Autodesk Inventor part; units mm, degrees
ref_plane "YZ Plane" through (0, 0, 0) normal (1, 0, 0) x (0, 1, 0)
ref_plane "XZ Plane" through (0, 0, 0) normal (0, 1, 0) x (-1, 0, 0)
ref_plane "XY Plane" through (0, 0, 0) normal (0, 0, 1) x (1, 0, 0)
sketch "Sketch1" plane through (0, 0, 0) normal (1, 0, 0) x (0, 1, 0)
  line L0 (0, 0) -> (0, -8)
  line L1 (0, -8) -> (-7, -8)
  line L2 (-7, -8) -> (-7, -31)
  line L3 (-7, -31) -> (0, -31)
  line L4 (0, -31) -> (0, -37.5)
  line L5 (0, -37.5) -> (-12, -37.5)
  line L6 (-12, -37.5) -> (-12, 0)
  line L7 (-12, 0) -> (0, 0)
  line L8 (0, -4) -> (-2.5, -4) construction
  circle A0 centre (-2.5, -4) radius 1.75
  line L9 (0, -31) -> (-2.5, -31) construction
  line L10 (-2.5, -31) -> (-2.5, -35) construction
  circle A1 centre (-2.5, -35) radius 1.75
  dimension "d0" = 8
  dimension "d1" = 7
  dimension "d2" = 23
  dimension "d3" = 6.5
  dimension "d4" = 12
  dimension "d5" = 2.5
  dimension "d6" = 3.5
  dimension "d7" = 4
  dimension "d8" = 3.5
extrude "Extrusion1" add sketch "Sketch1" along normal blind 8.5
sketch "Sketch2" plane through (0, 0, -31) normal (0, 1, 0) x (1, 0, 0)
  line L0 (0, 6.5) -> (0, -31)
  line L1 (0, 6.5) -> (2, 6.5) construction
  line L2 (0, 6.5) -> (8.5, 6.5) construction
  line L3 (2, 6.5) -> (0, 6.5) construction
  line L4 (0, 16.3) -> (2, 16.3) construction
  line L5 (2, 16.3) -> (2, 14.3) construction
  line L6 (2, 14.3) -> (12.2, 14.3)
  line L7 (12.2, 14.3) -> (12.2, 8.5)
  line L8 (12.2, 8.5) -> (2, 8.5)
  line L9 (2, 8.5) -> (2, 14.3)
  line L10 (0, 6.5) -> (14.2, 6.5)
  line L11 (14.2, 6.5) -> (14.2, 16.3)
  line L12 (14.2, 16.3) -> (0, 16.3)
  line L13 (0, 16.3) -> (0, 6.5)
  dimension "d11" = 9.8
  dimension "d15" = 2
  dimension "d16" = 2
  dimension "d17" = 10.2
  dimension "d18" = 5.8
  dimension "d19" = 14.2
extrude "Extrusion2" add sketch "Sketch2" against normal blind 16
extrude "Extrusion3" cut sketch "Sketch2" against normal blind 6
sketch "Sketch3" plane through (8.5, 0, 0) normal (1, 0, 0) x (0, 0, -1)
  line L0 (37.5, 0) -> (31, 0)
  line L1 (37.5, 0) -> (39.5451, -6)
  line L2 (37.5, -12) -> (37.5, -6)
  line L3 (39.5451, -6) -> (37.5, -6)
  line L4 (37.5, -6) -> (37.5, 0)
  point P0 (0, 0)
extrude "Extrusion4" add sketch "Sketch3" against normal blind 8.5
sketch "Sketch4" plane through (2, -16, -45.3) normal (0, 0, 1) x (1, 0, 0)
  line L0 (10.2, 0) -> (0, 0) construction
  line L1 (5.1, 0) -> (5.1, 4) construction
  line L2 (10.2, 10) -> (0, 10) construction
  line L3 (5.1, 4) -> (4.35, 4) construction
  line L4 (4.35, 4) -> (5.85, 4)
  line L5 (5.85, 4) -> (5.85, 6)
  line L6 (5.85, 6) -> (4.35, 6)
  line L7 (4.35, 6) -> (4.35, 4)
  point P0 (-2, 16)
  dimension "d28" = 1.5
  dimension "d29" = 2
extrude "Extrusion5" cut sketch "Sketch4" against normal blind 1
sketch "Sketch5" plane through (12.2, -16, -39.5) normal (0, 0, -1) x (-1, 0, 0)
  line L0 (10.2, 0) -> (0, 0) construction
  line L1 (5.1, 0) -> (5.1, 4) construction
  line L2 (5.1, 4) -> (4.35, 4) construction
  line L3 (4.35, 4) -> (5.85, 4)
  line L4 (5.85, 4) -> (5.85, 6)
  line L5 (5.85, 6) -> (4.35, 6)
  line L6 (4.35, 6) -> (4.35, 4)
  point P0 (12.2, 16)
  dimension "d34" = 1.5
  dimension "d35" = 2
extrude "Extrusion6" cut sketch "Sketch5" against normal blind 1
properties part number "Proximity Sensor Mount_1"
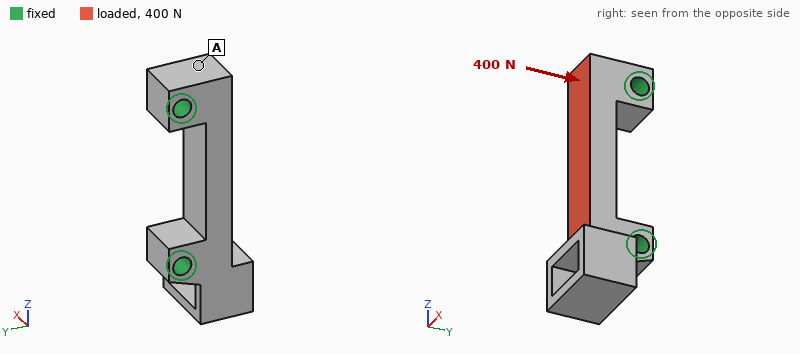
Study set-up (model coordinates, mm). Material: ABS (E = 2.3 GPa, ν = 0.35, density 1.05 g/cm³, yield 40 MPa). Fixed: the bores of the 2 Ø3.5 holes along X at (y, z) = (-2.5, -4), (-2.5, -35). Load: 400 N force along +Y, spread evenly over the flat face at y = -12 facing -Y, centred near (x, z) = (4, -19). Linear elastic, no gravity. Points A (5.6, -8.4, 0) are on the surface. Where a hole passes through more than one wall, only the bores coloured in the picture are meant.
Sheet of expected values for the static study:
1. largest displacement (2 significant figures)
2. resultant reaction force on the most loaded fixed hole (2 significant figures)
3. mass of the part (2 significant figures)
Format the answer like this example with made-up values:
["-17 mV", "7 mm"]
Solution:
["0.12 mm", "230 N", "3.3 g"]
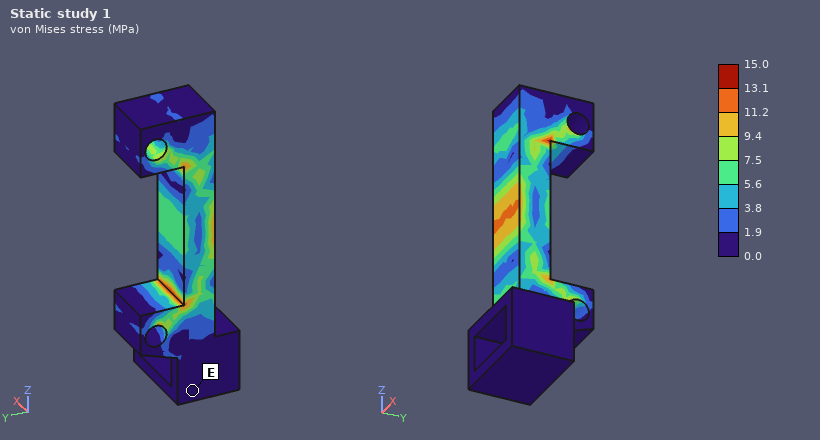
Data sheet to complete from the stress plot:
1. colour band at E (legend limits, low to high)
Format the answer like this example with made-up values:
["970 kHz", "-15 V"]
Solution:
["0.0 to 1.9 MPa"]
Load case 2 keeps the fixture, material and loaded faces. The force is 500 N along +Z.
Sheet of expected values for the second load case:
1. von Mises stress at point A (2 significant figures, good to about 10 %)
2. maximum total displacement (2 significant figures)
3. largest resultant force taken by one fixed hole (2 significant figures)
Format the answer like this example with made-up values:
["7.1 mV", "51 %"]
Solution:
["3.5 MPa", "0.15 mm", "260 N"]
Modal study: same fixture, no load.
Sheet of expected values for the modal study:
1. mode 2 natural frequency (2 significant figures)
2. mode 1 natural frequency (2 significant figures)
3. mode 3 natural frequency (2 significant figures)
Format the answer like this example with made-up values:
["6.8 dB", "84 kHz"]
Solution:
["3700 Hz", "3100 Hz", "6500 Hz"]
